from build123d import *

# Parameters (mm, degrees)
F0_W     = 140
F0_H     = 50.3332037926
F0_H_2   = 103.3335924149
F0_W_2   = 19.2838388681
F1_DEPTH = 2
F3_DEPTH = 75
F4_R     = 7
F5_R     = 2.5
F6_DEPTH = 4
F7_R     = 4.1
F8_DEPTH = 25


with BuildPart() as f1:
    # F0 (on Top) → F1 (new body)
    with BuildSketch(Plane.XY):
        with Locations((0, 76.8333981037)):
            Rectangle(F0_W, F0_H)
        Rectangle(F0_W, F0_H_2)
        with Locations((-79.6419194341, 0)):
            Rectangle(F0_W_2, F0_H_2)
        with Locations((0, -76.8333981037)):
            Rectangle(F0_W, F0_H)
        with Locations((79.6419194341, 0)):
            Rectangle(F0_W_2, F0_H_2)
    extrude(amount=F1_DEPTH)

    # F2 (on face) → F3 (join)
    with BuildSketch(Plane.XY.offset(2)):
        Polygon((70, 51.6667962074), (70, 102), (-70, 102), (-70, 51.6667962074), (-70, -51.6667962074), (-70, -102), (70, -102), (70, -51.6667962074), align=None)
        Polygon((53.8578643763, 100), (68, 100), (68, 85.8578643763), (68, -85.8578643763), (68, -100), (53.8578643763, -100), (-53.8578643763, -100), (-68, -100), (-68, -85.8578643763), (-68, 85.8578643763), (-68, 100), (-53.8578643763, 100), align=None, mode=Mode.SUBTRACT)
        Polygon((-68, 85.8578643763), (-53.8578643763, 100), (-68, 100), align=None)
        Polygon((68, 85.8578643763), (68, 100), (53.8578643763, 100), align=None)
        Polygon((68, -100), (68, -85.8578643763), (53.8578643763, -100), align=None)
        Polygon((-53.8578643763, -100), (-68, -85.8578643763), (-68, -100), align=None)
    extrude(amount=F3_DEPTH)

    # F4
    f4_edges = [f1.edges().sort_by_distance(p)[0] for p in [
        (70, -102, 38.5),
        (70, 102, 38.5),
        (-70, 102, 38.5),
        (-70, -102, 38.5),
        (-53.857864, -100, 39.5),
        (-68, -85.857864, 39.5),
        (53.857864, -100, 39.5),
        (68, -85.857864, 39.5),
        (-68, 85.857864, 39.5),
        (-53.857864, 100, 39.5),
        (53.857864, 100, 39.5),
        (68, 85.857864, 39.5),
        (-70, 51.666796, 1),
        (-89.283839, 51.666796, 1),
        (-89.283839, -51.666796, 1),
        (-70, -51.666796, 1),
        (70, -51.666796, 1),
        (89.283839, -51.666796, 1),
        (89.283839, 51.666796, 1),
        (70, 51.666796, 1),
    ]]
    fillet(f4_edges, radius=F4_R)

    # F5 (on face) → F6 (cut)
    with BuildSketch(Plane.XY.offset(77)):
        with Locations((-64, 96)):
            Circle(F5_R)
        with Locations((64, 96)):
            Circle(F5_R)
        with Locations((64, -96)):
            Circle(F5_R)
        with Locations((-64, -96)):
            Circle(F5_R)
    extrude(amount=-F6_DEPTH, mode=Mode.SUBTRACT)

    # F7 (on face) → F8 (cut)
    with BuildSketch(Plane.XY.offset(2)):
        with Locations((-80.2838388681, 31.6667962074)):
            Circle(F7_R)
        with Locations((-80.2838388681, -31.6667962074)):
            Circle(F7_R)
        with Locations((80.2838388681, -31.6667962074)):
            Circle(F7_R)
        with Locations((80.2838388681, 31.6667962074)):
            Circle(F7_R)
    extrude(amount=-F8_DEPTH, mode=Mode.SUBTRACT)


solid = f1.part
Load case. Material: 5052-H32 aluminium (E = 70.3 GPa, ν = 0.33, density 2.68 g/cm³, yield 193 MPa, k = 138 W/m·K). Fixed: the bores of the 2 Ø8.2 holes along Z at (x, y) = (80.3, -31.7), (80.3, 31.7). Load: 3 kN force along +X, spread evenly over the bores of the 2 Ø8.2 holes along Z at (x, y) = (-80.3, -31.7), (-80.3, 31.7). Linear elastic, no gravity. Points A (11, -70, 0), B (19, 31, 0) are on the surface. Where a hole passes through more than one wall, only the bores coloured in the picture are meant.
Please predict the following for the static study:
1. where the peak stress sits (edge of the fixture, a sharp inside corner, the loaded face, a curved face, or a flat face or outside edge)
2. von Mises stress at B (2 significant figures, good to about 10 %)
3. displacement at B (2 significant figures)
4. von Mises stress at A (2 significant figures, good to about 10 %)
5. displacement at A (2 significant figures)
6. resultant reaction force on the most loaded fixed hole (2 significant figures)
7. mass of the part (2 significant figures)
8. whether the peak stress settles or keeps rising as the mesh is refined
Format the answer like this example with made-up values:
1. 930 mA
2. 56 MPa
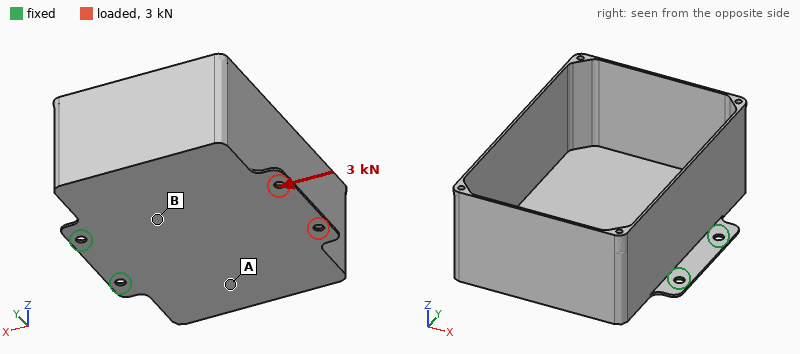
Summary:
1. a sharp inside corner
2. 12 MPa
3. 17 µm
4. 5.2 MPa
5. 21 µm
6. 1.5 kN
7. 520 g
8. keeps rising
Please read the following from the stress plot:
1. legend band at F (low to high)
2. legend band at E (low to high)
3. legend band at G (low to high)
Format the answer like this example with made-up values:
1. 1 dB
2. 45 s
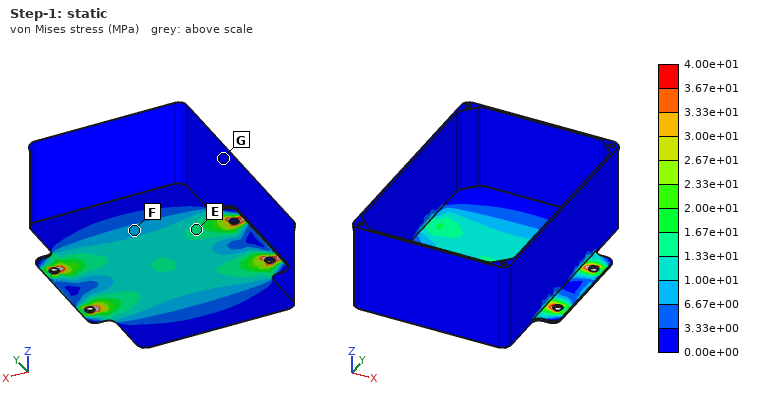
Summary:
1. 6.67e+00 to 1.00e+01 MPa
2. 1.33e+01 to 1.67e+01 MPa
3. 0.00e+00 to 3.33e+00 MPa
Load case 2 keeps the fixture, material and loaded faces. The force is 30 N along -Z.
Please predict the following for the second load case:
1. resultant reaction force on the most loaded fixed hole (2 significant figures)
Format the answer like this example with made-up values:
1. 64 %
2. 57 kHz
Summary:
1. 16 N
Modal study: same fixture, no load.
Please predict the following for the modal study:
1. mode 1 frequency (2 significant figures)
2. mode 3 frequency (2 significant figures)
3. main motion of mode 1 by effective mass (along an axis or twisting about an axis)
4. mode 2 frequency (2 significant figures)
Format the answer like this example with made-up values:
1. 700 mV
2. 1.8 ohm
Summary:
1. 36 Hz
2. 450 Hz
3. along Z
4. 94 Hz
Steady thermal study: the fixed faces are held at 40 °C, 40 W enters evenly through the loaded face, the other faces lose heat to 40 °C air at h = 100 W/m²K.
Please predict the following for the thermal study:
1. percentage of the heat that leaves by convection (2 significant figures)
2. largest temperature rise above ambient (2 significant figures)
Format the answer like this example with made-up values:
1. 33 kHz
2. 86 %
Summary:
1. 99 %
2. 44 K
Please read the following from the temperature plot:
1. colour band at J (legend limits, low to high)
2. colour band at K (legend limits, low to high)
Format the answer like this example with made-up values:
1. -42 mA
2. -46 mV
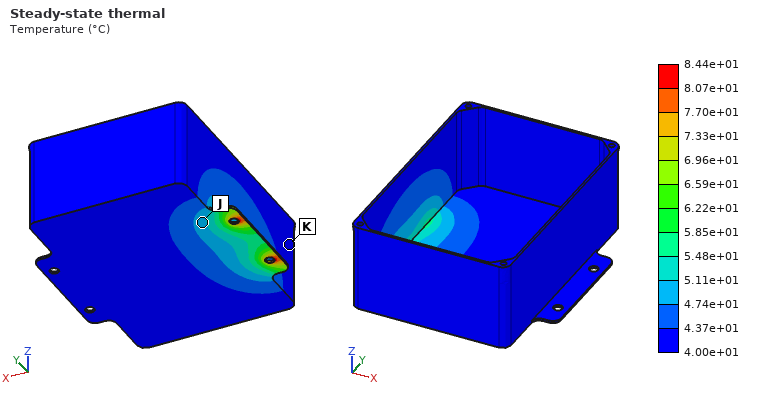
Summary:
1. 4.74e+01 to 5.11e+01 °C
2. 4.00e+01 to 4.37e+01 °C
